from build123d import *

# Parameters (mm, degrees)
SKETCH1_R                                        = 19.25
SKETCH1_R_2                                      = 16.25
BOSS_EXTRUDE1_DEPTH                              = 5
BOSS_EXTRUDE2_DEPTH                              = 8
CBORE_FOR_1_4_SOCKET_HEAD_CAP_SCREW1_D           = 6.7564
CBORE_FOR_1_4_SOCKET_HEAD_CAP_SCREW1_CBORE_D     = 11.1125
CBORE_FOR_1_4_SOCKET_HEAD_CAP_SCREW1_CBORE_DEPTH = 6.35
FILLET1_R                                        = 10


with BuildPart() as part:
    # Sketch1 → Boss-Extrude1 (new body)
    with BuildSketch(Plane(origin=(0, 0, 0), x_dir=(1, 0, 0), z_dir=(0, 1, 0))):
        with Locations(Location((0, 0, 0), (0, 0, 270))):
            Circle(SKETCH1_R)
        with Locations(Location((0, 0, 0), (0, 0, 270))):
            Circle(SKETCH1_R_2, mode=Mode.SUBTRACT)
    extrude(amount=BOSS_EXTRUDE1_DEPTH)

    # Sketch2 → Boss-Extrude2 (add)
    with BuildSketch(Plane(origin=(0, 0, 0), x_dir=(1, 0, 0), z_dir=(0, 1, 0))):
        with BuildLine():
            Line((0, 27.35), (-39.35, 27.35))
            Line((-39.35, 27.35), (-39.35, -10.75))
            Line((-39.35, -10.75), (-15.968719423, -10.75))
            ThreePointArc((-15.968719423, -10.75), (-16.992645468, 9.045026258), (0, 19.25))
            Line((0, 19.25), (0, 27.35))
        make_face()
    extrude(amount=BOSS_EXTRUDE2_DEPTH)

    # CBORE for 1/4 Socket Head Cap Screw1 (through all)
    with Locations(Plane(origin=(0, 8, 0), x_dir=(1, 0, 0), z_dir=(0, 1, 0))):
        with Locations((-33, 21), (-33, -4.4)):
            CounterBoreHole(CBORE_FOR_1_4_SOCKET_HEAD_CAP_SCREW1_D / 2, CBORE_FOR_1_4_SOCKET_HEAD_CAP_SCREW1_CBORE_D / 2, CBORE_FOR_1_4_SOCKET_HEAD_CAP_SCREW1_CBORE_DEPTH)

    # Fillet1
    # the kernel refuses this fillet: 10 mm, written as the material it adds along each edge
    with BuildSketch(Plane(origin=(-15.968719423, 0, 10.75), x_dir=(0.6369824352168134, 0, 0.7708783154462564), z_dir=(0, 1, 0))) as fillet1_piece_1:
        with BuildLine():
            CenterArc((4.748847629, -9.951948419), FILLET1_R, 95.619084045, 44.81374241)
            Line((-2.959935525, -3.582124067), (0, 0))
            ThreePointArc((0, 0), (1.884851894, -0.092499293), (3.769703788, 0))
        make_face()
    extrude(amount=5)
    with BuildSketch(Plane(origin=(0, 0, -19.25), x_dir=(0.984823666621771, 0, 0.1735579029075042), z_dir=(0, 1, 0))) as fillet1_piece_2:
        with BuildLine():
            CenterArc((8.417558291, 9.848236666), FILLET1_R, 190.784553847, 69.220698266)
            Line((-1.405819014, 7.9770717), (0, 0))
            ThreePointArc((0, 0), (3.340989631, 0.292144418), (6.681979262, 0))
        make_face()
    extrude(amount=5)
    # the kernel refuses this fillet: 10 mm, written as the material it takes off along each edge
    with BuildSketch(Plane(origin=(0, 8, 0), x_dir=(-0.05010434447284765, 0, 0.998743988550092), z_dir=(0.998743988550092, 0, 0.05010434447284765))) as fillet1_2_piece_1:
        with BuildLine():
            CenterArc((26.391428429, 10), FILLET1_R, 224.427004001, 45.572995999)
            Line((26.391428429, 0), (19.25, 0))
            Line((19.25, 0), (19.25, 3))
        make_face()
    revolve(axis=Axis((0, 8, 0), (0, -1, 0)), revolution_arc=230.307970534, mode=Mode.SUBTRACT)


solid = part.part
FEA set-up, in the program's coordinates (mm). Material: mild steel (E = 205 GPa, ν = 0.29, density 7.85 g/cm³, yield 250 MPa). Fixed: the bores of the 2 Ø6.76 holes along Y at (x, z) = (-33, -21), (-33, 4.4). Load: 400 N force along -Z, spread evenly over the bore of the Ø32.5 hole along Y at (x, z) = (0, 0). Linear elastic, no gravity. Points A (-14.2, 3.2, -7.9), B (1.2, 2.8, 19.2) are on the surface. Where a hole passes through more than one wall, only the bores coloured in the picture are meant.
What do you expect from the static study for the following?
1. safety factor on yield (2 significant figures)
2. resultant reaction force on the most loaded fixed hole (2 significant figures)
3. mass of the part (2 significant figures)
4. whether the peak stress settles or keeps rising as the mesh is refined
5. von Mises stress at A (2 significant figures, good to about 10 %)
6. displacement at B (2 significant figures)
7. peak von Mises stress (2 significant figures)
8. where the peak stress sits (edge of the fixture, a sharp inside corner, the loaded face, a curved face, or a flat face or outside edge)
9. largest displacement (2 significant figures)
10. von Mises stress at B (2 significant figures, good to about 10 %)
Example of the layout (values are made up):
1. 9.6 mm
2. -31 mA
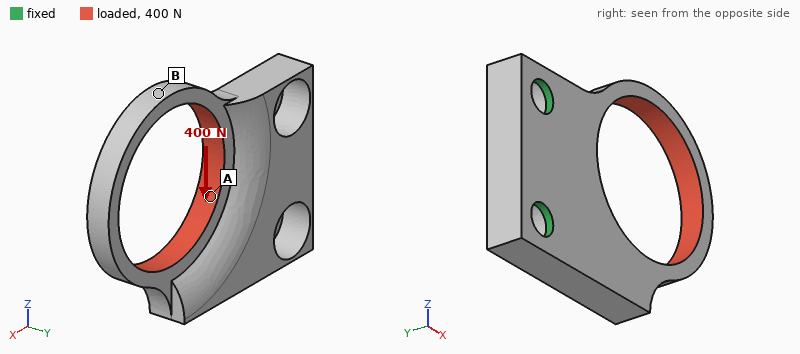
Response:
1. 2.7
2. 500 N
3. 64 g
4. settles
5. 16 MPa
6. 35 µm
7. 91 MPa
8. a curved face
9. 40 µm
10. 41 MPa
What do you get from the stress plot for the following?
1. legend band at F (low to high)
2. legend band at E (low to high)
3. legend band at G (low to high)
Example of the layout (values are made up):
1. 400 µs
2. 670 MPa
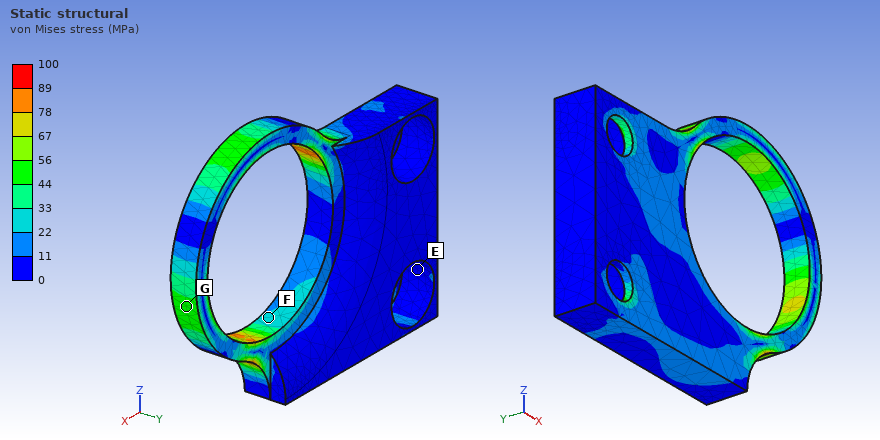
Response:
1. 22 to 33 MPa
2. 0 to 11 MPa
3. 44 to 56 MPa
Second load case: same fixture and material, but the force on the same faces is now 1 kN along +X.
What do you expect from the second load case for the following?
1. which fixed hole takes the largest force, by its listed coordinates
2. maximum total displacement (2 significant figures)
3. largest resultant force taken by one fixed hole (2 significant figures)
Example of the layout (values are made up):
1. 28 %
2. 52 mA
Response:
1. (-33, 4.4)
2. 58 µm
3. 780 N
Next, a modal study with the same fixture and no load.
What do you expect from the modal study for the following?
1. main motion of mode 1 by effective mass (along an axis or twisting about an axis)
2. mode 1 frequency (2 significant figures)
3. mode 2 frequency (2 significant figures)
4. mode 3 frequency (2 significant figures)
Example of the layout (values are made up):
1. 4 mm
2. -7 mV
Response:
1. along Y
2. 2100 Hz
3. 4400 Hz
4. 4500 Hz
